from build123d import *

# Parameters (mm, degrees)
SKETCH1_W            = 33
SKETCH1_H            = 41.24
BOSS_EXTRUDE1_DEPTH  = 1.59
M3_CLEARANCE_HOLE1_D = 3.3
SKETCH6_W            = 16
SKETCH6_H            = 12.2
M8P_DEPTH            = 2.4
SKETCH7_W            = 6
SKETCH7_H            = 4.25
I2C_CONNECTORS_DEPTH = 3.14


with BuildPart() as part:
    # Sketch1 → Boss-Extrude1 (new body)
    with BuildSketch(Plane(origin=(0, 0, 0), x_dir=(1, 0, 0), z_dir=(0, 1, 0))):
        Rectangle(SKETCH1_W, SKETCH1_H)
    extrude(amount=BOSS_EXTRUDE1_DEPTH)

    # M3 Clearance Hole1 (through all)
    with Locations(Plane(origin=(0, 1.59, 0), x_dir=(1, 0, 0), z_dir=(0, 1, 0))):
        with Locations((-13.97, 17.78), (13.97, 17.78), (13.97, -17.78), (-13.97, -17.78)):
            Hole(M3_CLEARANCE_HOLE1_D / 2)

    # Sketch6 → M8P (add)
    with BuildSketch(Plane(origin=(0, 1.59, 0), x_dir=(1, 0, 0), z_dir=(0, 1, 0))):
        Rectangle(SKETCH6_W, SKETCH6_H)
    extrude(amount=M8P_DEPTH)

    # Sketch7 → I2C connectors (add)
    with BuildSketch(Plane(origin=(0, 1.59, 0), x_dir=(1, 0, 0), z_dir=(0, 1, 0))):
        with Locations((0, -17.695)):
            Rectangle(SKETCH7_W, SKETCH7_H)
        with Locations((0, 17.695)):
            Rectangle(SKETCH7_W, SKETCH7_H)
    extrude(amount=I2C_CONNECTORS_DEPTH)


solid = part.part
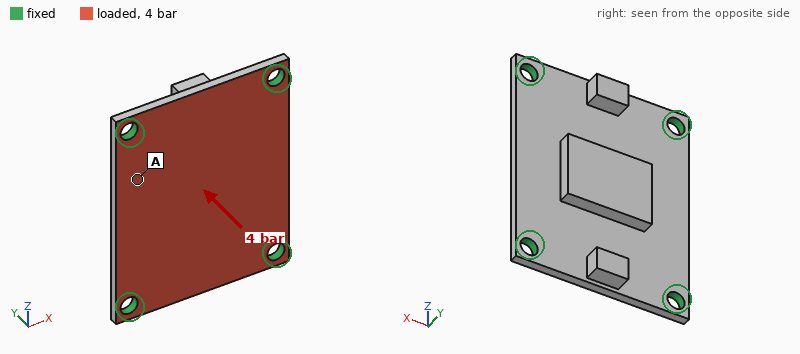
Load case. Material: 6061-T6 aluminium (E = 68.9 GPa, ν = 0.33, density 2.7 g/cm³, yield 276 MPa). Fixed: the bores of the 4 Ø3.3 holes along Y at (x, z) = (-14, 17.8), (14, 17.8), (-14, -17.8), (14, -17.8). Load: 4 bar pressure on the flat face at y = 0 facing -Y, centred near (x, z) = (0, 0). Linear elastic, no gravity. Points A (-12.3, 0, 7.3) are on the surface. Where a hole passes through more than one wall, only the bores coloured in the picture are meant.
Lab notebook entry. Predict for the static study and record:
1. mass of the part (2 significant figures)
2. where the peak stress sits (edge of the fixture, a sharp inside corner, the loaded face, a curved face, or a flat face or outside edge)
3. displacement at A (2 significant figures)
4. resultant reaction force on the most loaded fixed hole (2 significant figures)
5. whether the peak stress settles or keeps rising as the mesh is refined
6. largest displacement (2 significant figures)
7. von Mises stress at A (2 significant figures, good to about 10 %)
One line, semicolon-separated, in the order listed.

7.4 g; edge of the fixture; 47 µm; 140 N; keeps rising; 63 µm; 37 MPa
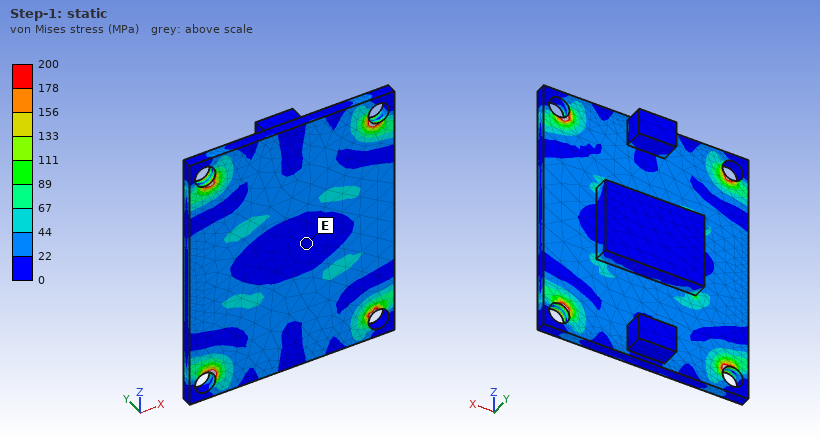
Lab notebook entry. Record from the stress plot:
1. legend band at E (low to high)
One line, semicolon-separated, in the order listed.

0 to 22 MPa
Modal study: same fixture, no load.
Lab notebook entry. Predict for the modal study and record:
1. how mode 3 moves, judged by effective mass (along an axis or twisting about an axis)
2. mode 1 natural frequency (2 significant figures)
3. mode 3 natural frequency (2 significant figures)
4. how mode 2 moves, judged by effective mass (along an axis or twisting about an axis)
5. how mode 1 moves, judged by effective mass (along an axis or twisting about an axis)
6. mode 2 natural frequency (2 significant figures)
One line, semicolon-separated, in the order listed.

twisting about X; 5600 Hz; 11 kHz; twisting about Z; along Y; 8800 Hz
